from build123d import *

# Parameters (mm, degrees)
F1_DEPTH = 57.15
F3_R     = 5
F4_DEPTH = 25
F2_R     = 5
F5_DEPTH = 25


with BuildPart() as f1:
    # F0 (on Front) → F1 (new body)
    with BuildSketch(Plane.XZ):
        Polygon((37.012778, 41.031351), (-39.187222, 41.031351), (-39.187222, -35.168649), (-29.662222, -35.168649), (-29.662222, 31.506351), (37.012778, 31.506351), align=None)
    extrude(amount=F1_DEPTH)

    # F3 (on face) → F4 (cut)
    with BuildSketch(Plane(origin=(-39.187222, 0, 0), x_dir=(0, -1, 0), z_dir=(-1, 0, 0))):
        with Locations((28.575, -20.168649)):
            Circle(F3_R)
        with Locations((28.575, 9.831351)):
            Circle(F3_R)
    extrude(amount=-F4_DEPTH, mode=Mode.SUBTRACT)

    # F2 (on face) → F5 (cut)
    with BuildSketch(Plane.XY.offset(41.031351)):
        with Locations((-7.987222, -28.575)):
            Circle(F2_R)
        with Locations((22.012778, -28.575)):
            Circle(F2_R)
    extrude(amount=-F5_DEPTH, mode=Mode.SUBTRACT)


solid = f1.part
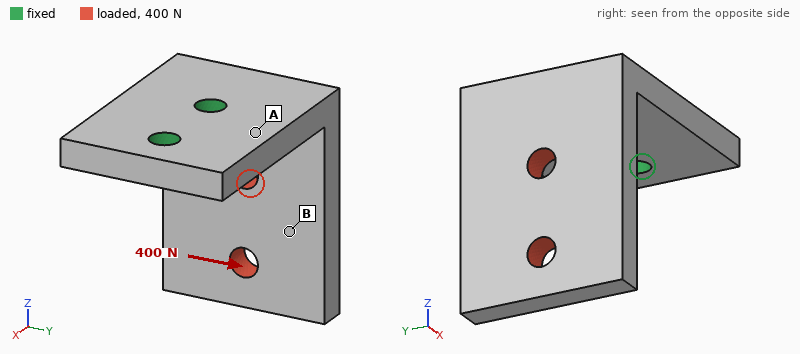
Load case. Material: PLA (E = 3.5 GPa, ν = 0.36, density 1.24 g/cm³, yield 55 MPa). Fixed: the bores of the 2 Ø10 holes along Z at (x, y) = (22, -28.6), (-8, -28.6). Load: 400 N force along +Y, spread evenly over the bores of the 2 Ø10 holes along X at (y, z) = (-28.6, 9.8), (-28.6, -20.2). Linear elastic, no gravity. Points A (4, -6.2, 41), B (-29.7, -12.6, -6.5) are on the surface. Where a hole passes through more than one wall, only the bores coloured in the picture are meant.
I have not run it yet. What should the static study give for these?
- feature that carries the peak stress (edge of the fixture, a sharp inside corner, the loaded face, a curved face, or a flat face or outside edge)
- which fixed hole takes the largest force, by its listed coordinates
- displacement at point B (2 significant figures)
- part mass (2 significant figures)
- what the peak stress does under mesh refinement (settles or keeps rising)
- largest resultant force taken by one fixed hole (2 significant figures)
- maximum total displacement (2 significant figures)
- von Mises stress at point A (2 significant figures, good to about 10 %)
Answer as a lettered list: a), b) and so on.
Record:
a) edge of the fixture
b) (-8, -28.6)
c) 0.85 mm
d) 93 g
e) keeps rising
f) 620 N
g) 1.4 mm
h) 6.9 MPa
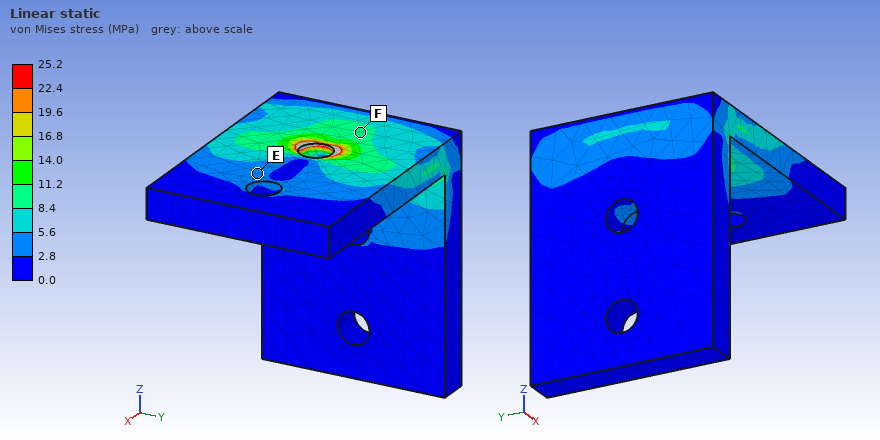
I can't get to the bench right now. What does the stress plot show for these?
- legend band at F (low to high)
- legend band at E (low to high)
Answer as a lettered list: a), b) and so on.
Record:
a) 8.4 to 11.2 MPa
b) 2.8 to 5.6 MPa
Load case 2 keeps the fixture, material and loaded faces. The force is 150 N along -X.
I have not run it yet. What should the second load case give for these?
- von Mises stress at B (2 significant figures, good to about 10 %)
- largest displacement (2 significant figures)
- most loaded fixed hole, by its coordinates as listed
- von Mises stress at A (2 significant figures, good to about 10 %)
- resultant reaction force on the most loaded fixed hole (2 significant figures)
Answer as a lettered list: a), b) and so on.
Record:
a) 1.4 MPa
b) 1.3 mm
c) (-8, -28.6)
d) 1.3 MPa
e) 150 N
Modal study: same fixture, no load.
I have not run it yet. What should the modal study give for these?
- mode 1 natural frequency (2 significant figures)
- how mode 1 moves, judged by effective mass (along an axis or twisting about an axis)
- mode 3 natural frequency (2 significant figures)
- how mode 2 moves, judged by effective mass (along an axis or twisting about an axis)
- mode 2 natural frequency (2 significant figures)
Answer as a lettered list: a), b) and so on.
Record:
a) 330 Hz
b) along X
c) 1200 Hz
d) along Y
e) 500 Hz
